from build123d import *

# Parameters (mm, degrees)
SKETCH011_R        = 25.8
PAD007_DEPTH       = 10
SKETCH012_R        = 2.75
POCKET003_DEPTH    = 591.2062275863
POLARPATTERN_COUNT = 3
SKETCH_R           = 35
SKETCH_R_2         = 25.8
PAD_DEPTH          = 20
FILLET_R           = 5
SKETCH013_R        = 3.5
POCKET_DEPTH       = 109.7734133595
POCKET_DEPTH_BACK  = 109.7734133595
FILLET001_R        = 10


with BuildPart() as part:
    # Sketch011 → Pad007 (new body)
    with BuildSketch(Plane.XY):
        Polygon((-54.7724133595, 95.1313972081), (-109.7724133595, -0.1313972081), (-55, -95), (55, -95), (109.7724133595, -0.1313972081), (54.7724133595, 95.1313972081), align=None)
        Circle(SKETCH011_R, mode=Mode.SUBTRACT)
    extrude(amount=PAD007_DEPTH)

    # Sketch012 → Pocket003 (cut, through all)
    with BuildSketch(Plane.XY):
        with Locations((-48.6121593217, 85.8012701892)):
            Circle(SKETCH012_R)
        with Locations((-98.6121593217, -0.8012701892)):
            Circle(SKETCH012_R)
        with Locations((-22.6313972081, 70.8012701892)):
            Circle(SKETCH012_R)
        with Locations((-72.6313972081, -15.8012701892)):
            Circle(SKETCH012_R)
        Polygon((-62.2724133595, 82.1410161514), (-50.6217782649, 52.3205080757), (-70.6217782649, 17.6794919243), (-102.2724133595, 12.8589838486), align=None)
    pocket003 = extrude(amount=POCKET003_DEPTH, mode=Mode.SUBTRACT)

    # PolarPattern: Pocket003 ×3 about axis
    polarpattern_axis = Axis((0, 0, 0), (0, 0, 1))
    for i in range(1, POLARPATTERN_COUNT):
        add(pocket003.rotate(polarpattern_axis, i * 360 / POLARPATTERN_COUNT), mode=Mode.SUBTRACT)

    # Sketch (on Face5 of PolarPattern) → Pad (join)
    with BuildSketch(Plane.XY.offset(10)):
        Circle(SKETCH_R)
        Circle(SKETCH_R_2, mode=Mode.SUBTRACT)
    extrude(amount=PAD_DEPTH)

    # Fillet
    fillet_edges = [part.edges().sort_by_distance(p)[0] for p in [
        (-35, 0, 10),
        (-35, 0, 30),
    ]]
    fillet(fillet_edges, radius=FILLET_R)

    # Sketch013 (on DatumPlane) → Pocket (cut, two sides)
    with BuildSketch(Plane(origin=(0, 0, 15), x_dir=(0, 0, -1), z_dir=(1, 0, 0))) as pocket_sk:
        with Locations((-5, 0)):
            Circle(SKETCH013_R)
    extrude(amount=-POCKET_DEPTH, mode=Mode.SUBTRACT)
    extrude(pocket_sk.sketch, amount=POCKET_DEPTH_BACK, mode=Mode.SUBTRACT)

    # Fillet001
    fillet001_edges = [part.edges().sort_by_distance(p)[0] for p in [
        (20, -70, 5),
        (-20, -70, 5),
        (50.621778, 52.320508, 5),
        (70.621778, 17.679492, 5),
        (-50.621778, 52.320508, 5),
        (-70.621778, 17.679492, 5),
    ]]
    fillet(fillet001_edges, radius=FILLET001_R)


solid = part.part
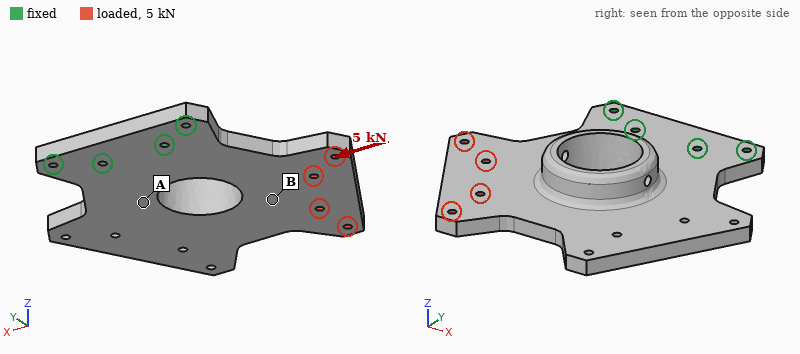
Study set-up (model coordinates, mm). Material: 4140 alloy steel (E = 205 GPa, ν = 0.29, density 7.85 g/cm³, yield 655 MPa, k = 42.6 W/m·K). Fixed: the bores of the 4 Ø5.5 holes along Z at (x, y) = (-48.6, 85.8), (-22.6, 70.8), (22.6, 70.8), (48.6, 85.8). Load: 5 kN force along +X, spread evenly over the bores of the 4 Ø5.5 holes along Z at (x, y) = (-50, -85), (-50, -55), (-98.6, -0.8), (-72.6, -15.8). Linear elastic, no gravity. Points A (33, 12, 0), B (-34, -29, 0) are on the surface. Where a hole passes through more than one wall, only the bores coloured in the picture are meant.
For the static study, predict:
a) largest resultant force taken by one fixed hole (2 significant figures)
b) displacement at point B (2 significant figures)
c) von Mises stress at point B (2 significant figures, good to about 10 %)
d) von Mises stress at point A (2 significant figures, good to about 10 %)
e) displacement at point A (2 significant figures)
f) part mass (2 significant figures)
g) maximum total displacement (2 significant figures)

4.3 kN
27 µm
6.2 MPa
17 MPa
13 µm
2.2 kg
46 µm
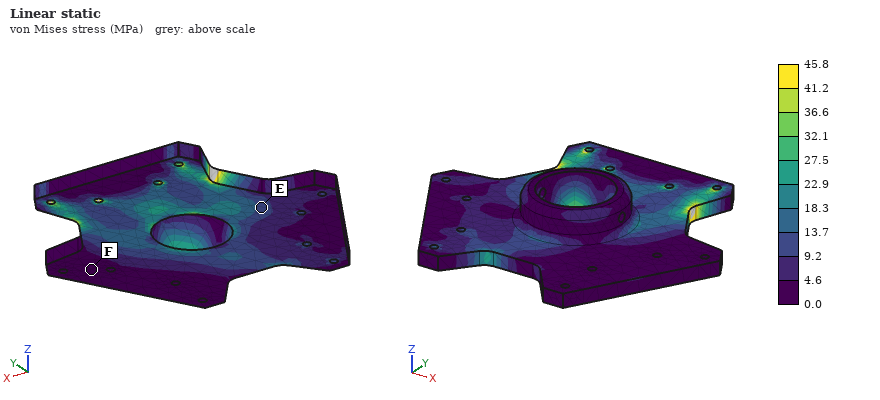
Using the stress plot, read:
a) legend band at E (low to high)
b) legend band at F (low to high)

9.2 to 13.7 MPa
0.0 to 4.6 MPa
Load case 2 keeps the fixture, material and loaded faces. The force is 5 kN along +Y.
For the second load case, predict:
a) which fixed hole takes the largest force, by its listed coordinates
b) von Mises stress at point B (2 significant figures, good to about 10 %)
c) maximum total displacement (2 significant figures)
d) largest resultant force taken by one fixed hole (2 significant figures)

(-22.6, 70.8)
8.9 MPa
26 µm
3.9 kN
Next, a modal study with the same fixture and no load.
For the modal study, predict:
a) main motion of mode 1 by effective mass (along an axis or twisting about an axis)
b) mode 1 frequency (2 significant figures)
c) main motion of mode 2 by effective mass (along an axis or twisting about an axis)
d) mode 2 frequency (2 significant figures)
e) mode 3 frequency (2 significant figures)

along Z
300 Hz
twisting about Y
650 Hz
1600 Hz
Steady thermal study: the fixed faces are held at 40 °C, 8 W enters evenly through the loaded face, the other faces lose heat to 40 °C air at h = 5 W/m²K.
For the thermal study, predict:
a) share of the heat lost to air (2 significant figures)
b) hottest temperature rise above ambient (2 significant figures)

33 %
20 K
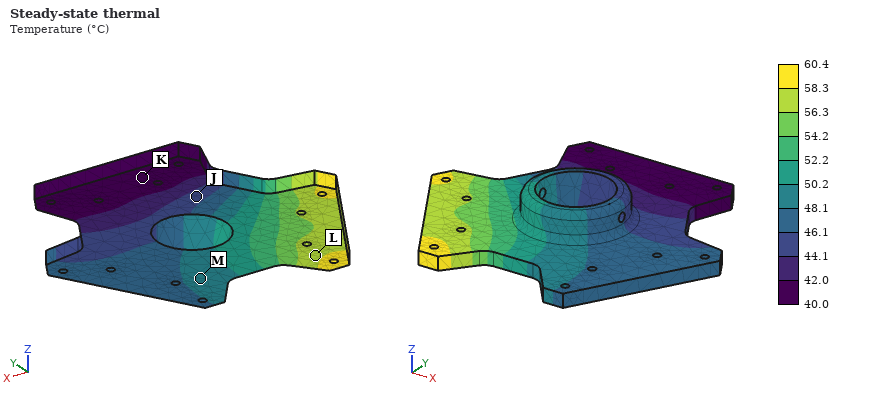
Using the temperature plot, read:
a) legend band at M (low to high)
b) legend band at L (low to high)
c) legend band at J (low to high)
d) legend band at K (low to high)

48.1 to 50.2 °C
56.3 to 58.3 °C
44.1 to 46.1 °C
40.0 to 42.0 °C
